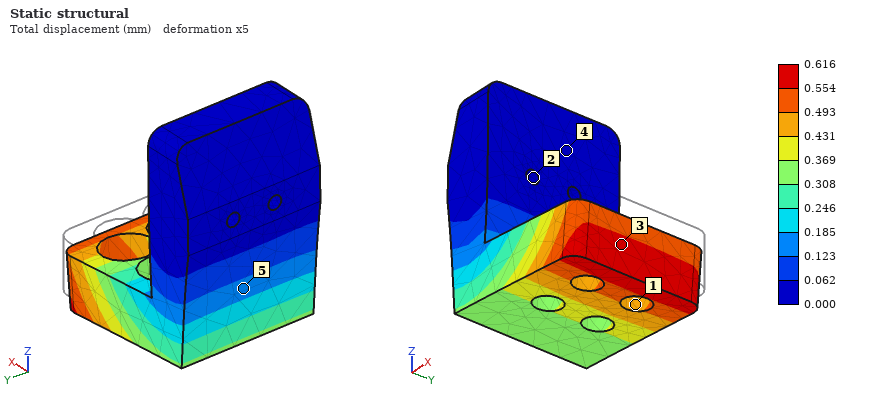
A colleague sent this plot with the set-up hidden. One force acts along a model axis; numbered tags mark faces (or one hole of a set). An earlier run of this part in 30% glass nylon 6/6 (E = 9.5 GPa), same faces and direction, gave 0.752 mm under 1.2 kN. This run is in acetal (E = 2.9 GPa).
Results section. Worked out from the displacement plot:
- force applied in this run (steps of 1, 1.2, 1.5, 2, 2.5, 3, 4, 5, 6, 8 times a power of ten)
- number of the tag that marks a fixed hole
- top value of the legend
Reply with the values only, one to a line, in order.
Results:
300 N
2
0.616 mm
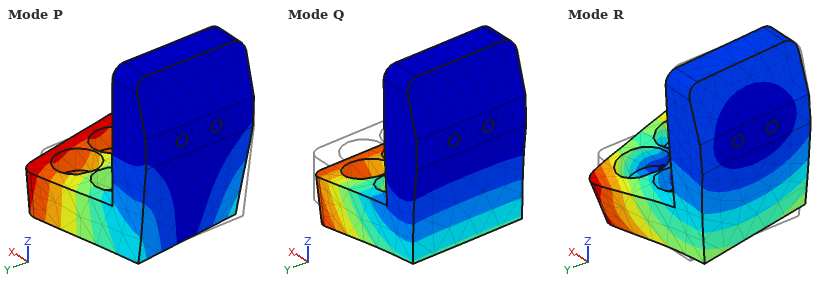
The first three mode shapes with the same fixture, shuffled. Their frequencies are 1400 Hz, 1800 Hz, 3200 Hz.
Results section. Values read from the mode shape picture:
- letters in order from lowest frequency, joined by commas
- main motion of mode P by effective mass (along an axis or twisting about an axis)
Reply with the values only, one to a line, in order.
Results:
Q, P, R
along Y
